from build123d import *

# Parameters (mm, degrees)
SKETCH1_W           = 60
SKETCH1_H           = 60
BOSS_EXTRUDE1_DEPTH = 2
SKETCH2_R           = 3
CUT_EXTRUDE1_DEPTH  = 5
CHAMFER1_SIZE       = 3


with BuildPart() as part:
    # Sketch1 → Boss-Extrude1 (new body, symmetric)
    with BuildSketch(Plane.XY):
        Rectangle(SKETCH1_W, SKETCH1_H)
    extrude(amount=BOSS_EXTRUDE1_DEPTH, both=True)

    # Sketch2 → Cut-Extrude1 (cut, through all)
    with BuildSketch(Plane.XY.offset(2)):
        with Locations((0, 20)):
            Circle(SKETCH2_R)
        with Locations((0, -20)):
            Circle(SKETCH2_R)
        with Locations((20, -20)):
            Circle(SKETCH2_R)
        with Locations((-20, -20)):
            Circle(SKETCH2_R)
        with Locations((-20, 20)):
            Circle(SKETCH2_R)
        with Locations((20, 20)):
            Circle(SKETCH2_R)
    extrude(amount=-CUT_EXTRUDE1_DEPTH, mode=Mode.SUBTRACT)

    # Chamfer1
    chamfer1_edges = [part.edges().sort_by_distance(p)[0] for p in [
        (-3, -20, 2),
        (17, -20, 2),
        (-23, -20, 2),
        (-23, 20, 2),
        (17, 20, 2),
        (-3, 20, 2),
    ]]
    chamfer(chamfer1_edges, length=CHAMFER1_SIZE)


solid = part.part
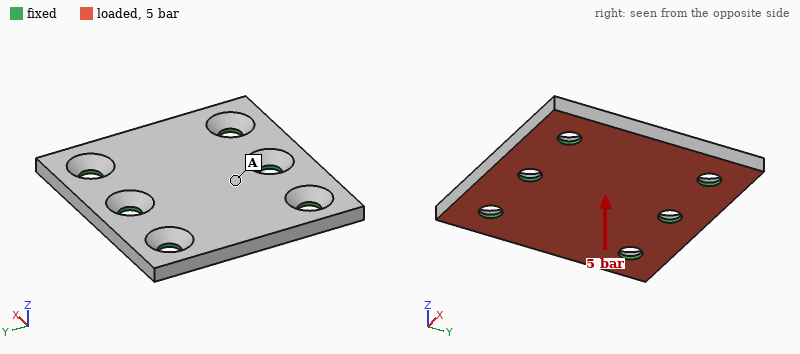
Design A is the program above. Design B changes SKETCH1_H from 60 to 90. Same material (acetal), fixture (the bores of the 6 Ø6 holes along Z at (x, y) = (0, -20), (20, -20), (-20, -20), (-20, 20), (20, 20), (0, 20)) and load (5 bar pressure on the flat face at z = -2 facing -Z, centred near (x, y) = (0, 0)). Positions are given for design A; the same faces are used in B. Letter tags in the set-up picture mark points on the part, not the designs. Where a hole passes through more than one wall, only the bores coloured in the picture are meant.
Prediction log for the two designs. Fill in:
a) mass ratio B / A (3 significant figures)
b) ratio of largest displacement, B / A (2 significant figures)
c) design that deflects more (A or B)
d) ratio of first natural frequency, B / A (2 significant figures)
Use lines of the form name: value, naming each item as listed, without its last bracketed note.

mass ratio B / A: 1.55
ratio of largest displacement, B / A: 5.8
design that deflects more: B
ratio of first natural frequency, B / A: 0.40
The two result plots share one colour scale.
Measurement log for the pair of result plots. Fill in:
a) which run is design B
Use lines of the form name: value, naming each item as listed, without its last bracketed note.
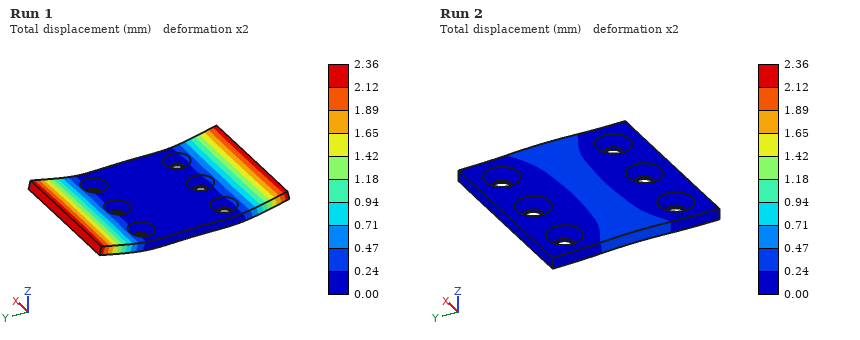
which run is design B: Run 1
